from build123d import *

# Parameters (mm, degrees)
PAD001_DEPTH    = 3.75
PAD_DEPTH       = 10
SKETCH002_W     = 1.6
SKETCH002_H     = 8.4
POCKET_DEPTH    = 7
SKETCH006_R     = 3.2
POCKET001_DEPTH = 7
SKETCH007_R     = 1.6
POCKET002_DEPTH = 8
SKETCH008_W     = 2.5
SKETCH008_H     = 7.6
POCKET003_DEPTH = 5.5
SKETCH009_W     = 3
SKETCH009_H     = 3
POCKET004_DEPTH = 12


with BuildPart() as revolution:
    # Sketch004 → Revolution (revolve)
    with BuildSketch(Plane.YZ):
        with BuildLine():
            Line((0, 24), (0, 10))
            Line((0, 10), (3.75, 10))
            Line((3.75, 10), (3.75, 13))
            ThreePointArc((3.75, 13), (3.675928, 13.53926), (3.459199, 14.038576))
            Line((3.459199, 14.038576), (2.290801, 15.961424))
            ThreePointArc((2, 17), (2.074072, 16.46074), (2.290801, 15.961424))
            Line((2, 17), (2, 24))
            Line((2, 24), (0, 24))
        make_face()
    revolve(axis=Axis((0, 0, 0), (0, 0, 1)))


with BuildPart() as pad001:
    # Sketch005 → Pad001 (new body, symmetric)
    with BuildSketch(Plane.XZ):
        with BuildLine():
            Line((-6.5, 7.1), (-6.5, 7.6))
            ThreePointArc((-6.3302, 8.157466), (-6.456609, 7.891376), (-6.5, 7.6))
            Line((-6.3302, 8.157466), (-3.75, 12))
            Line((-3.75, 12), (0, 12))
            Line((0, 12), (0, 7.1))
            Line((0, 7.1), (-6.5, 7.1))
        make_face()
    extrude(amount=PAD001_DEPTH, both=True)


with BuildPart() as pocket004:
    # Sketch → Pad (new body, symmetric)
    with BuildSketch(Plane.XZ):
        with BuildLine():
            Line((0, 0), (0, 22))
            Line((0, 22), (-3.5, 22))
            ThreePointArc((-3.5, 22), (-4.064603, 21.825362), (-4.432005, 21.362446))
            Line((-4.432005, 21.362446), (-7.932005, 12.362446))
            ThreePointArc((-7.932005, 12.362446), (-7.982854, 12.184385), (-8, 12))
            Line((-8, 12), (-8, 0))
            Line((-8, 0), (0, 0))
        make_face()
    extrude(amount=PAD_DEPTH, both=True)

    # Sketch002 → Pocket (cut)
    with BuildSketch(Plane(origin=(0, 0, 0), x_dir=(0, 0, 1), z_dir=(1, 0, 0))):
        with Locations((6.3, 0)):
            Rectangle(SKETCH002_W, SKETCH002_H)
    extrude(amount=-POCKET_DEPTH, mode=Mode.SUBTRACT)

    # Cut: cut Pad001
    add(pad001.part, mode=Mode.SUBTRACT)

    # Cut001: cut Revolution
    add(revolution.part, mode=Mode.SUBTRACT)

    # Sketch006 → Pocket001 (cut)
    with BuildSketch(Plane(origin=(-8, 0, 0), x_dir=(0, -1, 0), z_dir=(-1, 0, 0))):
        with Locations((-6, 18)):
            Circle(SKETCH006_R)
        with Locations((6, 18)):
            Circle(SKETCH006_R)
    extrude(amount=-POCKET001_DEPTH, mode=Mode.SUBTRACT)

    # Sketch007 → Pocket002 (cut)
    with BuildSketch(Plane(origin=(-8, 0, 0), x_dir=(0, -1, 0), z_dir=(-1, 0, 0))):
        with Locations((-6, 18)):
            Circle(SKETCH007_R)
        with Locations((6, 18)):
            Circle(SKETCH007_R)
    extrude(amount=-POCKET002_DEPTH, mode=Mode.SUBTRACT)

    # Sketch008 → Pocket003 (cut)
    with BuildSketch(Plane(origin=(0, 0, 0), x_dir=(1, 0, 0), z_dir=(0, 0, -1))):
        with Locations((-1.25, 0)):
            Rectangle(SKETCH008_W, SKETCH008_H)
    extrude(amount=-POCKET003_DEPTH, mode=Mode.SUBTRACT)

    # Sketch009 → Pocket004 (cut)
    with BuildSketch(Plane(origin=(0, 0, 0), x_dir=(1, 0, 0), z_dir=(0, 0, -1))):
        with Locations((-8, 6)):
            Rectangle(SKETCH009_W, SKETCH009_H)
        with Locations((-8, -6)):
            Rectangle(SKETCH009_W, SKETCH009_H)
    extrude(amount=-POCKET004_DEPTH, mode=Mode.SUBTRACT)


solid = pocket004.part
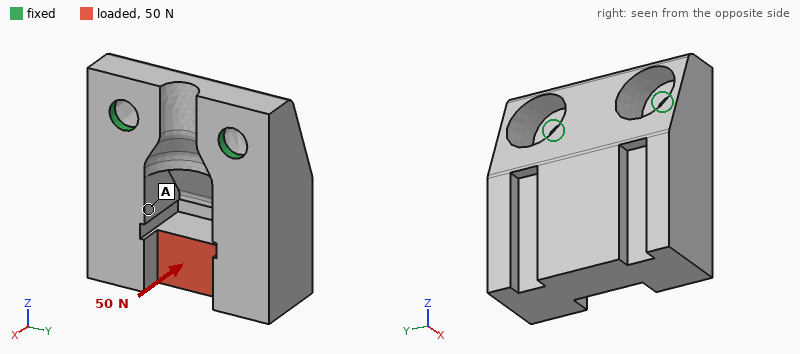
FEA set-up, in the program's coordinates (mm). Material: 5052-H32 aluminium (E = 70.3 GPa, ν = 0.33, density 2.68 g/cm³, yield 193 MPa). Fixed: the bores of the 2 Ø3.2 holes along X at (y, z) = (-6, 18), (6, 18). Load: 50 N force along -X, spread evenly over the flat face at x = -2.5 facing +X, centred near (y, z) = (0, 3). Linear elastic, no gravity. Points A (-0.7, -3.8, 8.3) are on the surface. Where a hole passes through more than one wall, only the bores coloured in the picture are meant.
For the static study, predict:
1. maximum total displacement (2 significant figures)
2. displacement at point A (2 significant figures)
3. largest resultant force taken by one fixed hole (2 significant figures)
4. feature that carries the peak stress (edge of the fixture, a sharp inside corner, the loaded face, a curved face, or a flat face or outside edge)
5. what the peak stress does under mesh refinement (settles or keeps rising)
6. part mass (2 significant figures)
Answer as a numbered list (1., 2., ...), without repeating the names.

1. 33 µm
2. 16 µm
3. 25 N
4. edge of the fixture
5. keeps rising
6. 5.9 g
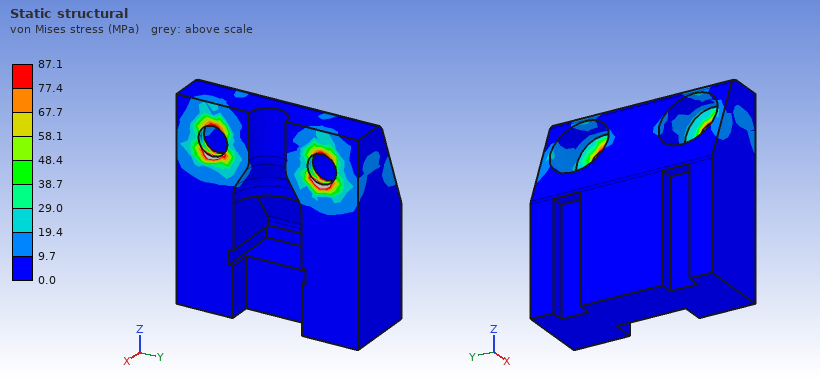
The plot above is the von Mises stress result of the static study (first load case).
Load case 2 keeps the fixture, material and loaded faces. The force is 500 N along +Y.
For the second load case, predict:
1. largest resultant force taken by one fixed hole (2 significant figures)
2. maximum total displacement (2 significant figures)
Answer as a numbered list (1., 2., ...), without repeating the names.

1. 530 N
2. 44 µm
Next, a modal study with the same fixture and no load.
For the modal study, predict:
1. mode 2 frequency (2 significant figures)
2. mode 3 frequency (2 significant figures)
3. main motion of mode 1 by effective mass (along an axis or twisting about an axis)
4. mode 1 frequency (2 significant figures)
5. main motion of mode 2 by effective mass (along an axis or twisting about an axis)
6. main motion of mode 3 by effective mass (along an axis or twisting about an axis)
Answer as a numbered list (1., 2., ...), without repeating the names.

1. 12 kHz
2. 16 kHz
3. along X
4. 4000 Hz
5. along Y
6. along Y
